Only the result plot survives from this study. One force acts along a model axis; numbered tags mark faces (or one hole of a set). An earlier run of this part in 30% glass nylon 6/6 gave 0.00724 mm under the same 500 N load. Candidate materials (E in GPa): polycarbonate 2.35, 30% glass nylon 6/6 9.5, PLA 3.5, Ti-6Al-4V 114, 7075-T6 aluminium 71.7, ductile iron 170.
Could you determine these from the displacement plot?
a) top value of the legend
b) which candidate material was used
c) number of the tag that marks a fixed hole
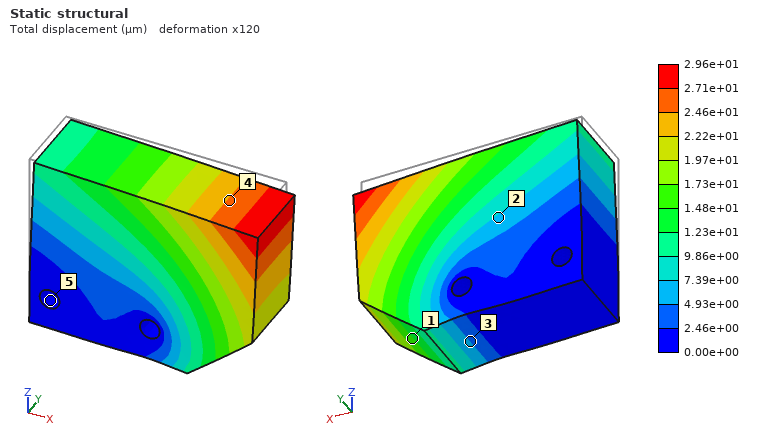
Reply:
2.96e+01 µm
polycarbonate
5
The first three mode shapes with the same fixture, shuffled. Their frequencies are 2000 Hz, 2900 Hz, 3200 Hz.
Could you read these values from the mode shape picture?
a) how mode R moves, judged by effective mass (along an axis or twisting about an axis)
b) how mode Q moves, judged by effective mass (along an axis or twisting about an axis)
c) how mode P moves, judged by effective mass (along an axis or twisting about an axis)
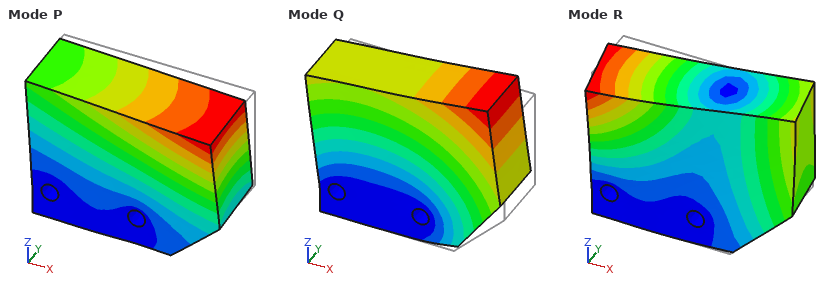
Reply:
twisting about Z
along X
along Y
